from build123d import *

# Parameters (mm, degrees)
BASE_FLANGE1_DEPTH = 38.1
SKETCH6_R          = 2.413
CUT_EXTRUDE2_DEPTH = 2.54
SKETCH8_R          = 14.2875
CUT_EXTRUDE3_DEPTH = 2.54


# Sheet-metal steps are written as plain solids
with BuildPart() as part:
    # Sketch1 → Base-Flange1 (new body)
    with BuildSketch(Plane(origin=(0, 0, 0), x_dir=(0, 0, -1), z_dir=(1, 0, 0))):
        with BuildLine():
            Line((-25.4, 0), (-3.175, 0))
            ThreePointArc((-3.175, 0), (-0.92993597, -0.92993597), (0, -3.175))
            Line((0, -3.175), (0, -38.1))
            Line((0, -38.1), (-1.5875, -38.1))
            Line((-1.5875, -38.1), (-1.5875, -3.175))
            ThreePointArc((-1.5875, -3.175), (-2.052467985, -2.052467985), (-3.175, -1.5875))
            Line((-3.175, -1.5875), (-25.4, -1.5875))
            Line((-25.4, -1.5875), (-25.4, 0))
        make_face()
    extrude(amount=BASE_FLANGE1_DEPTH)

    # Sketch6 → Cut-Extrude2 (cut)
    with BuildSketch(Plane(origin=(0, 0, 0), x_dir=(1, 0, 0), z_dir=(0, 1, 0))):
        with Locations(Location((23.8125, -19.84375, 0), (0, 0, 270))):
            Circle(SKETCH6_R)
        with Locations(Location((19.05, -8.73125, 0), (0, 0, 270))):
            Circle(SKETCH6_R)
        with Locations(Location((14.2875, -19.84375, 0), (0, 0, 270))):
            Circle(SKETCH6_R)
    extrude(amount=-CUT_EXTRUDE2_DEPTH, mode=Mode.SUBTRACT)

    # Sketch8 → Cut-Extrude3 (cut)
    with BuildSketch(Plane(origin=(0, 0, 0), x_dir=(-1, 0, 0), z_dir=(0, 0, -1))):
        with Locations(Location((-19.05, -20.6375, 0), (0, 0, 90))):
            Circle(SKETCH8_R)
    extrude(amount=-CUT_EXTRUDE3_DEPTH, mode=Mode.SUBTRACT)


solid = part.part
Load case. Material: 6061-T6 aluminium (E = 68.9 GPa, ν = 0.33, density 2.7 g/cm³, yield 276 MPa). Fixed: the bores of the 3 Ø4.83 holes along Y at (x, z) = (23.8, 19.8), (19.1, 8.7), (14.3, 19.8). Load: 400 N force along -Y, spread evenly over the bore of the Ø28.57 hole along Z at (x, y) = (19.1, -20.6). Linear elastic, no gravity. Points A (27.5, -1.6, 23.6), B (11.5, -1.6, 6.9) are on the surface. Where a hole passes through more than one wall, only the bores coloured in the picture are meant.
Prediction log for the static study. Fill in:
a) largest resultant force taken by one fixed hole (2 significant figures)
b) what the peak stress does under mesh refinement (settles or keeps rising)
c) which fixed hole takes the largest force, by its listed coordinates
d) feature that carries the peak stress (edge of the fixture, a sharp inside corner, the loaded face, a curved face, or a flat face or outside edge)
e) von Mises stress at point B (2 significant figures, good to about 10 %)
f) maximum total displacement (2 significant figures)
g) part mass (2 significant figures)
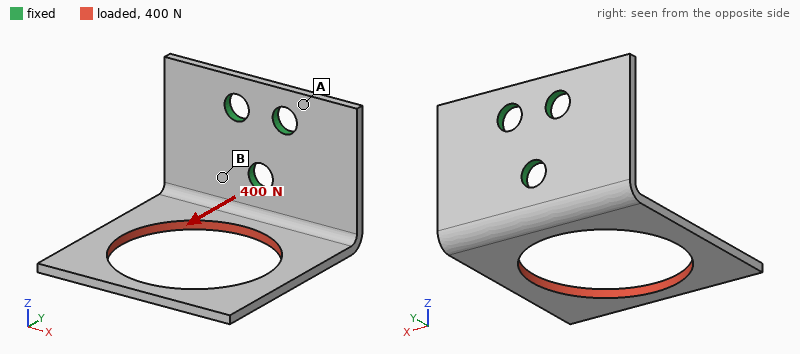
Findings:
480 N
keeps rising
(19.1, 8.7)
edge of the fixture
89 MPa
0.52 mm
7.0 g
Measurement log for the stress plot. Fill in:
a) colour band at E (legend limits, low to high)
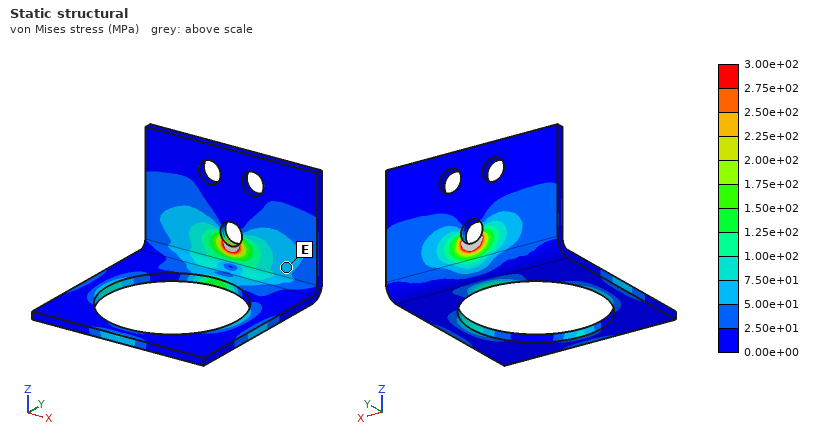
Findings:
5.00e+01 to 7.50e+01 MPa
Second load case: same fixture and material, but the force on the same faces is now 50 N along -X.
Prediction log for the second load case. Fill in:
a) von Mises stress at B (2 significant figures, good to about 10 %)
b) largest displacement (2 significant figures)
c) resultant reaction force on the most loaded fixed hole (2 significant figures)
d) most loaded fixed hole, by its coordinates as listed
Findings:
22 MPa
0.22 mm
51 N
(19.1, 8.7)
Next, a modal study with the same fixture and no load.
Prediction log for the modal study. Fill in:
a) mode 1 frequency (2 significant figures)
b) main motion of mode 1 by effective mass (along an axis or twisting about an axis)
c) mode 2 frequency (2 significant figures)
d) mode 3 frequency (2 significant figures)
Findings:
700 Hz
along Z
1400 Hz
1800 Hz
